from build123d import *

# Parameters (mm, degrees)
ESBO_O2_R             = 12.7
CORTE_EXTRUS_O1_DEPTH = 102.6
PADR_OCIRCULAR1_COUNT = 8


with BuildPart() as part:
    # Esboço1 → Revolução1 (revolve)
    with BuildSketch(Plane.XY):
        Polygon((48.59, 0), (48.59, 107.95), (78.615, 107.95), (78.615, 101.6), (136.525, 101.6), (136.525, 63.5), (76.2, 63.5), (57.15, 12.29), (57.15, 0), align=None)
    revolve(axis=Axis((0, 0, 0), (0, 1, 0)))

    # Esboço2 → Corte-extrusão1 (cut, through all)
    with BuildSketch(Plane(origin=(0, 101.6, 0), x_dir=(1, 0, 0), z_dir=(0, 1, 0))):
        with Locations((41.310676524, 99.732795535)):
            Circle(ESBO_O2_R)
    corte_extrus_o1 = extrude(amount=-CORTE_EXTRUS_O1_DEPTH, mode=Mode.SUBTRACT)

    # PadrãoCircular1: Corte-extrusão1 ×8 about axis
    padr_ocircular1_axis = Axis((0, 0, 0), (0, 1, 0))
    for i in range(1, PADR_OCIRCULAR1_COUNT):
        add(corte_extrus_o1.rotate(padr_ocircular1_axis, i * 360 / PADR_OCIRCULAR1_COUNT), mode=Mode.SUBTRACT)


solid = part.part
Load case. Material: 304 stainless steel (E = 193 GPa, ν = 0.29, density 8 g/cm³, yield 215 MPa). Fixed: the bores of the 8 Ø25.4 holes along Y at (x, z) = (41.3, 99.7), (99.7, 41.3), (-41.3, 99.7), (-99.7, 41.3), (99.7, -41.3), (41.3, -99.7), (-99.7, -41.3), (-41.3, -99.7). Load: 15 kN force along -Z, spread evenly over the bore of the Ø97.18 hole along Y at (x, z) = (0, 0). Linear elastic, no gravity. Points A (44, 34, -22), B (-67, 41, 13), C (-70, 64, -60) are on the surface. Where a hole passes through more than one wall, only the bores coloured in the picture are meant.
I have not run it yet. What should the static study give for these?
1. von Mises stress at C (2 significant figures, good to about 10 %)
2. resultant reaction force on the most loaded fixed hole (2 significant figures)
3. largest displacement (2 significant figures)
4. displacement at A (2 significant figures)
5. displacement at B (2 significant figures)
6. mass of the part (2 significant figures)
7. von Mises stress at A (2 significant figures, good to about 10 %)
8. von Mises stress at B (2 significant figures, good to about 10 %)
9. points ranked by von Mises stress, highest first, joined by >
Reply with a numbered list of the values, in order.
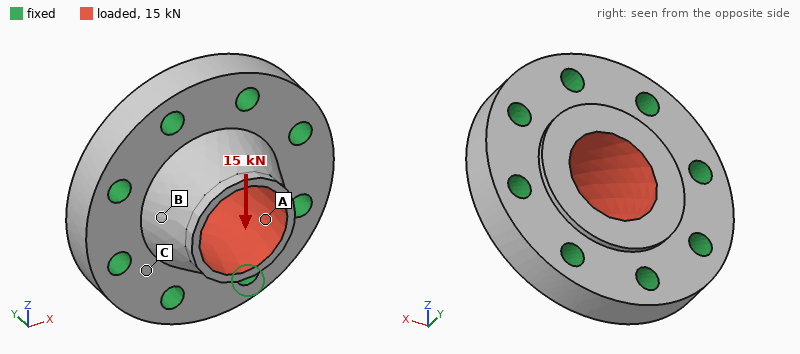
1. 0.67 MPa
2. 2.8 kN
3. 2.4 µm
4. 1.0 µm
5. 0.69 µm
6. 18 kg
7. 2.9 MPa
8. 1.6 MPa
9. A > B > C
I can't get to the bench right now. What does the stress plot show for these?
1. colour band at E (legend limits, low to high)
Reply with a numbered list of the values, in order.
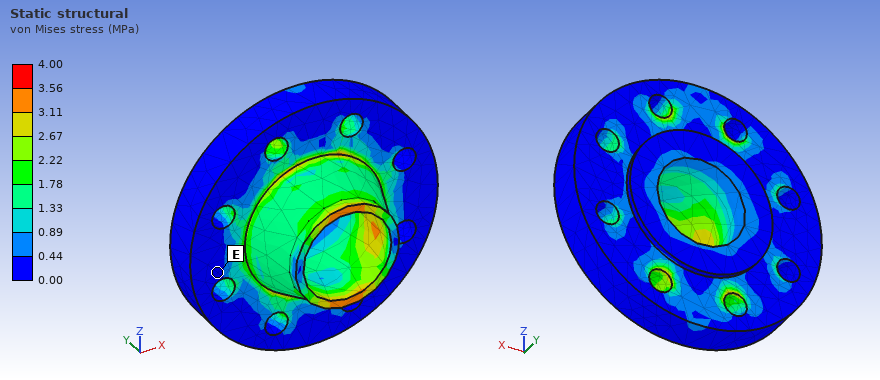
1. 0.00 to 0.44 MPa
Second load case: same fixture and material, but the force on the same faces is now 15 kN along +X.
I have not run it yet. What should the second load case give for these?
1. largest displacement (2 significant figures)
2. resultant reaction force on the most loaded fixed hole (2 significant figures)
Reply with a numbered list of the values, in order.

1. 2.4 µm
2. 2.8 kN
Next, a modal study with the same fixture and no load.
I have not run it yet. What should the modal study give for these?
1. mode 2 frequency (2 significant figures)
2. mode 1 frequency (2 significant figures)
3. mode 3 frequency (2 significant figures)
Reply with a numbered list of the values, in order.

1. 7900 Hz
2. 7800 Hz
3. 7900 Hz
